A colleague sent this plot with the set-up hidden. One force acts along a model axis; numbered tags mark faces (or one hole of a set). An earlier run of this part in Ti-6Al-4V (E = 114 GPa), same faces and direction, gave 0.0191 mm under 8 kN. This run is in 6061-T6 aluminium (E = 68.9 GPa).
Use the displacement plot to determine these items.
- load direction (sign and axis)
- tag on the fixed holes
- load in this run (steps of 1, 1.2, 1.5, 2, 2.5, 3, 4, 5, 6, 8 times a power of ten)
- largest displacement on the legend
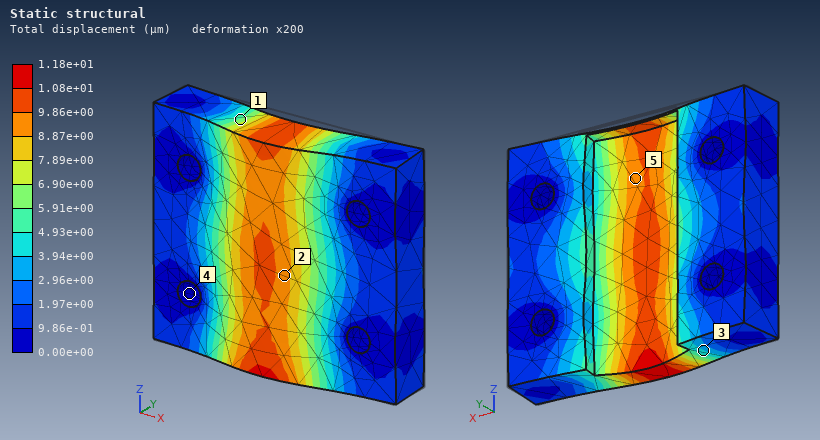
-Y
4
3 kN
1.18e+01 µm
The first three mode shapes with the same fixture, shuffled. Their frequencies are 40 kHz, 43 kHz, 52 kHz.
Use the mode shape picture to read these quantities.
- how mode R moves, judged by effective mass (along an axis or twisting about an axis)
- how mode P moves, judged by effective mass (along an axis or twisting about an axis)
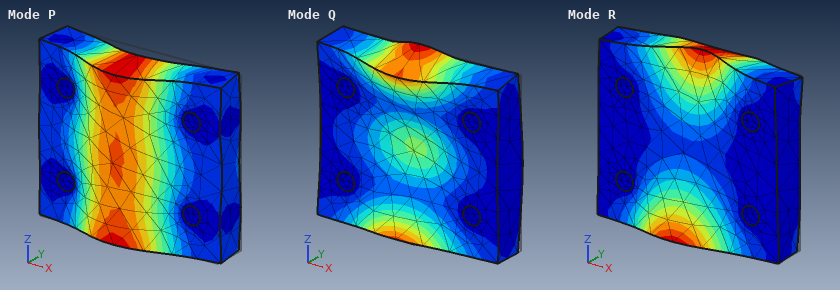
twisting about X
along Y
